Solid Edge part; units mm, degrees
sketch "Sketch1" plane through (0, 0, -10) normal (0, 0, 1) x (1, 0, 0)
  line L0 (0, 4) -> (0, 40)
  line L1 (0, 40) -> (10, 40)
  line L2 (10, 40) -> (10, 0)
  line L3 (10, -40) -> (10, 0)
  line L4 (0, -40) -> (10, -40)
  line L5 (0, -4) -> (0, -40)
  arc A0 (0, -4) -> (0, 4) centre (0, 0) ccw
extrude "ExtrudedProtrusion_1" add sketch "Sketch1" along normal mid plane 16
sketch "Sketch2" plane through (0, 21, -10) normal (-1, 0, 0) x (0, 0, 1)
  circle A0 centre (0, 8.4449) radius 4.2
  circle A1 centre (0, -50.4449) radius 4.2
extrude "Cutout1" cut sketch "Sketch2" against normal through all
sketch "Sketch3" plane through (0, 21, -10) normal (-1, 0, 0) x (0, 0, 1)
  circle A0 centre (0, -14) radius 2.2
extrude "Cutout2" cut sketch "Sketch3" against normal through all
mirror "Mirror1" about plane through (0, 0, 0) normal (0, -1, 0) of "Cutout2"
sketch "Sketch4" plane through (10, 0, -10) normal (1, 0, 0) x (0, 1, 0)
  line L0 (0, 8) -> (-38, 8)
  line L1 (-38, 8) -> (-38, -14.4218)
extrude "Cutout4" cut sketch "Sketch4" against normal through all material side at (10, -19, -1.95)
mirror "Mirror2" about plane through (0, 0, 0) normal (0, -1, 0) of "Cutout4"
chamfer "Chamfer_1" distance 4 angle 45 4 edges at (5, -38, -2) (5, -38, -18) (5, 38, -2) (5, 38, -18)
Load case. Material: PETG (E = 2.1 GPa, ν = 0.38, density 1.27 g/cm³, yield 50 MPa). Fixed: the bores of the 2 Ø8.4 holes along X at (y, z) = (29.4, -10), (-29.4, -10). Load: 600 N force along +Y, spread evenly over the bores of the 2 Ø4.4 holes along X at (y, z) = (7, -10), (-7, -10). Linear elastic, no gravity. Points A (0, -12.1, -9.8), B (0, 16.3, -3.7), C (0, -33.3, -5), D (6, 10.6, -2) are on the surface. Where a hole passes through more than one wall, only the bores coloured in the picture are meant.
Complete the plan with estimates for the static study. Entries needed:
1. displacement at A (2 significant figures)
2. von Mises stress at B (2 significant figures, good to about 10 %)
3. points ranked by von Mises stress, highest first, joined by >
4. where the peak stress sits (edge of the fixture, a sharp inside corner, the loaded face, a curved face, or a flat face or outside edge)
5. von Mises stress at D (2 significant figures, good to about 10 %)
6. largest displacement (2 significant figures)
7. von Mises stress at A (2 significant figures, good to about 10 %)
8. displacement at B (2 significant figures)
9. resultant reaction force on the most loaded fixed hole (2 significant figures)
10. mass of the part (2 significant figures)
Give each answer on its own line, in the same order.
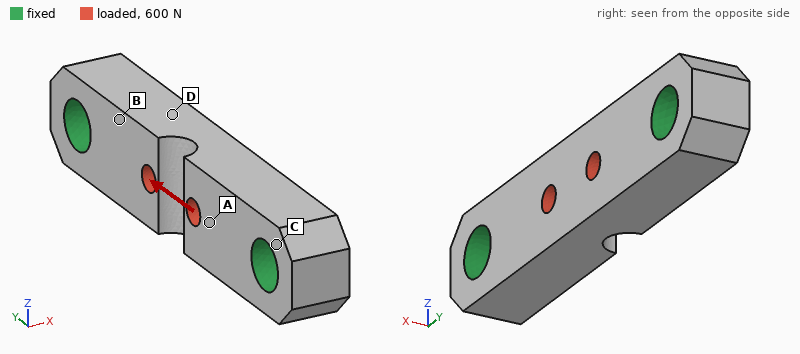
15 µm
1.7 MPa
A > B > D > C
a curved face
1.1 MPa
38 µm
2.5 MPa
11 µm
300 N
13 g
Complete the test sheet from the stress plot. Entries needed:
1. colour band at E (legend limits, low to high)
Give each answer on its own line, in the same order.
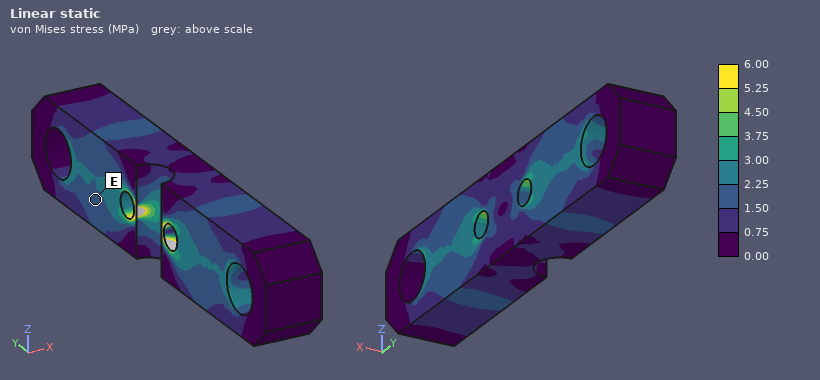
1.50 to 2.25 MPa
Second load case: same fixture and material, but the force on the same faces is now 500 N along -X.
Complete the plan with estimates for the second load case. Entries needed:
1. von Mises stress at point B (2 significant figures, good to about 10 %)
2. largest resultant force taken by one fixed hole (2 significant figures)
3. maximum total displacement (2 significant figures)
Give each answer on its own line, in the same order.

4.6 MPa
280 N
0.23 mm
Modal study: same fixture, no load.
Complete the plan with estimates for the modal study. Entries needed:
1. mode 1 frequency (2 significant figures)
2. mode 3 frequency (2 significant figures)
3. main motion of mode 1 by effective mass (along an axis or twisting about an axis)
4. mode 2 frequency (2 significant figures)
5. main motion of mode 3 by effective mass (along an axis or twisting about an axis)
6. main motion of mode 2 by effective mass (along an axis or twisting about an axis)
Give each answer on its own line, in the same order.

3700 Hz
6500 Hz
along X
4500 Hz
twisting about Y
along Z
